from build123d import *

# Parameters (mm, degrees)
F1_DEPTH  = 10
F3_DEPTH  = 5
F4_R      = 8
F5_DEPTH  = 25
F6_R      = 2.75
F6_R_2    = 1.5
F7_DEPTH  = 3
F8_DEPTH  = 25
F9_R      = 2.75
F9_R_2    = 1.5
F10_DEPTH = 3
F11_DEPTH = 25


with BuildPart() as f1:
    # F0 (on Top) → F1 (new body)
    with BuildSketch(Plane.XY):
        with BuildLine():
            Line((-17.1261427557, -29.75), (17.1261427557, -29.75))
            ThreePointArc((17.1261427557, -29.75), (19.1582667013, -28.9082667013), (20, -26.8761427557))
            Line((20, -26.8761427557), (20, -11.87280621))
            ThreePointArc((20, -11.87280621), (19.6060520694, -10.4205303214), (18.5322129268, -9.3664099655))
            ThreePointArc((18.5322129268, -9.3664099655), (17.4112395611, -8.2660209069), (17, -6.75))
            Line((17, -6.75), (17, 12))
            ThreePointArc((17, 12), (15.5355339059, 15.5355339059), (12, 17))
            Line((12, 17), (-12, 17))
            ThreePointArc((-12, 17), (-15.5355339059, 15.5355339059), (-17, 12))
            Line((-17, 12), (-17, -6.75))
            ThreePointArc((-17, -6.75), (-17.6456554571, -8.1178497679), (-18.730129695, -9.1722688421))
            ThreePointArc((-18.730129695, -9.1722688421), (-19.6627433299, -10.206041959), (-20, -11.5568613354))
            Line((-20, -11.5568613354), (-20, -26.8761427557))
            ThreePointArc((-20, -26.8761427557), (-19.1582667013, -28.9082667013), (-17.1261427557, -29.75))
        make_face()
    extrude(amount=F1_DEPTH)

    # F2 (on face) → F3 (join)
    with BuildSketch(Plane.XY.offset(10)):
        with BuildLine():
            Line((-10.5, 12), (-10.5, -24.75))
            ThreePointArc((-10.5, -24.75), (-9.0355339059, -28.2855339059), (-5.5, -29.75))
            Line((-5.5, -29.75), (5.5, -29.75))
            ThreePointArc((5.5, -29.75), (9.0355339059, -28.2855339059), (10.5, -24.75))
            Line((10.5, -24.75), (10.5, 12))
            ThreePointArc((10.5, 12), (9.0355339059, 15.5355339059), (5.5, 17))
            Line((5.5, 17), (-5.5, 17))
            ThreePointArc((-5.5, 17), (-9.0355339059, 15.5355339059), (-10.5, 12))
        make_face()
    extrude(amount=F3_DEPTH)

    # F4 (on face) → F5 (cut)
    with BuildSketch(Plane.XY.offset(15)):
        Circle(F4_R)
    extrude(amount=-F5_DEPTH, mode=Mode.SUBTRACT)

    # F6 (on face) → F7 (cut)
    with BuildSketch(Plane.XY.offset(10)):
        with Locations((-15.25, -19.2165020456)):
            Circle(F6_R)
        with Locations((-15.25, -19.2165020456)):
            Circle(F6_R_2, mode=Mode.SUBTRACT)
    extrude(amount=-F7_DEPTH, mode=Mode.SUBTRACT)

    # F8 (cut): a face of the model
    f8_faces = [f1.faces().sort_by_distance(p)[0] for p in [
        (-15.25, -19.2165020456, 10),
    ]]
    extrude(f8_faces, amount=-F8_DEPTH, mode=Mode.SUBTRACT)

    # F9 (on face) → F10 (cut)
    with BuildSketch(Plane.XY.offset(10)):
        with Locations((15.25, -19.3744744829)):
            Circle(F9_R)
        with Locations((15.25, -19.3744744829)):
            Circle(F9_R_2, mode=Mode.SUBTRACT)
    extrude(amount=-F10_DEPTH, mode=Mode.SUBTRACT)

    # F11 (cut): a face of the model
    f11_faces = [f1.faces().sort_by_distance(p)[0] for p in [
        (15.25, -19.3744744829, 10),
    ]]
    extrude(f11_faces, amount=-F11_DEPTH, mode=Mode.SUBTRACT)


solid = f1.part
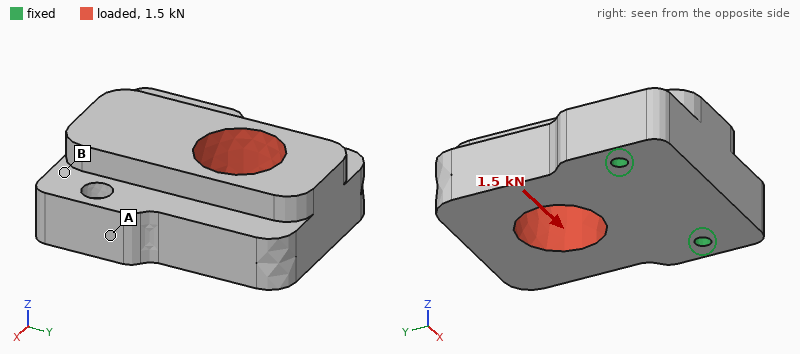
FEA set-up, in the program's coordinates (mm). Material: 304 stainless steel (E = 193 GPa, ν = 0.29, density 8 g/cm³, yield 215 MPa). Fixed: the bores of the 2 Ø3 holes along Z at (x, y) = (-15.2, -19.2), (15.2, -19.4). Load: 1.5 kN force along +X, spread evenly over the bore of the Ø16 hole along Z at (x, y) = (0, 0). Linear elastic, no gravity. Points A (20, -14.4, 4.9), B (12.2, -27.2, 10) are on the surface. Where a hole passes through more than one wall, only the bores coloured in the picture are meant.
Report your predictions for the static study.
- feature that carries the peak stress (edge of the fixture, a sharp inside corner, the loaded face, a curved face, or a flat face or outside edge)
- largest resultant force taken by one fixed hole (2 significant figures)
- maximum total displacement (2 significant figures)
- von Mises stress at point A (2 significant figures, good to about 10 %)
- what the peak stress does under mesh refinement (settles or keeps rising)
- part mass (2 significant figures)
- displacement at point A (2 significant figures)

edge of the fixture
1.2 kN
4.0 µm
6.9 MPa
keeps rising
150 g
0.82 µm
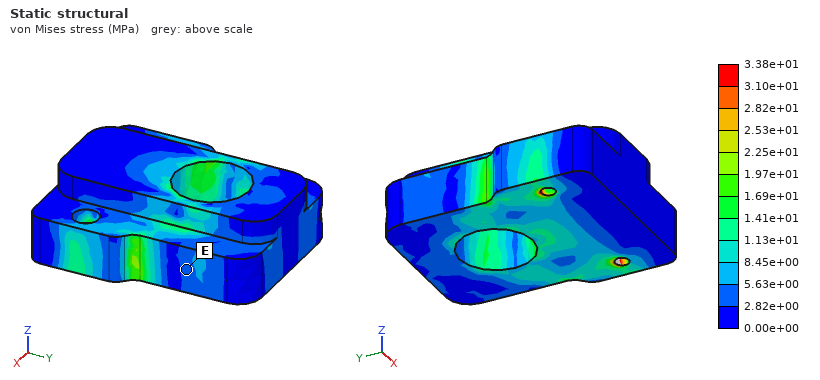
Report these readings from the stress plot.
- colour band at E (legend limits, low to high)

2.82e+00 to 5.63e+00 MPa
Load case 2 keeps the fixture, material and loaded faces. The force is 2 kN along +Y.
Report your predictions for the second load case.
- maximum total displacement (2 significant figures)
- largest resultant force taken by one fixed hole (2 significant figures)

8.7 µm
1.0 kN
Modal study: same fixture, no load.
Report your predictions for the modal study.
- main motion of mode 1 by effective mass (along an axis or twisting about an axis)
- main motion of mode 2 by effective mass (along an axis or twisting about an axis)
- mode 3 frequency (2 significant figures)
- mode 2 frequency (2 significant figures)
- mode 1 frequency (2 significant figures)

along Z
along X
13 kHz
11 kHz
4000 Hz
